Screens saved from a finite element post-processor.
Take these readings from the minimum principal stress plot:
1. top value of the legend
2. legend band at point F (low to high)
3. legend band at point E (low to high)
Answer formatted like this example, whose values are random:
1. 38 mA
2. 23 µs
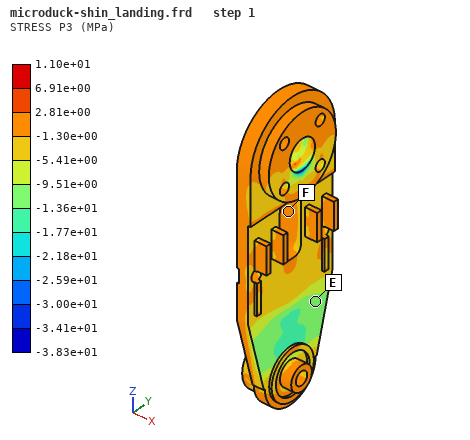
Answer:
1. 1.10e+01 MPa
2. -1.30e+00 to 2.81e+00 MPa
3. -1.36e+01 to -9.51e+00 MPa
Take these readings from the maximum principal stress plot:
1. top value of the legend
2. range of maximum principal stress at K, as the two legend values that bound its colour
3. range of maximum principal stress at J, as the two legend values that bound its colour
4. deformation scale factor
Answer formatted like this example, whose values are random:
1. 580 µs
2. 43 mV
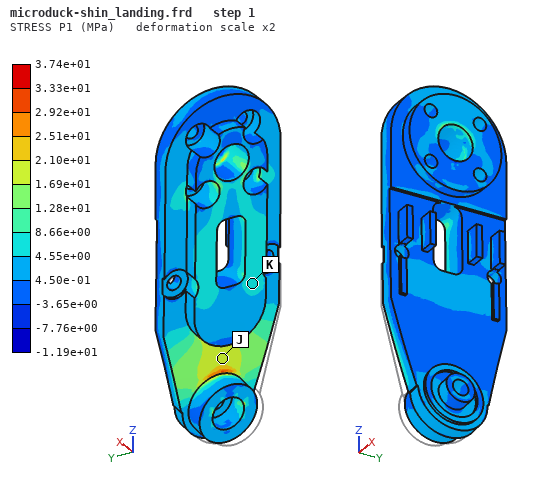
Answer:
1. 3.74e+01 MPa
2. 4.55e+00 to 8.66e+00 MPa
3. 1.69e+01 to 2.10e+01 MPa
4. 2
